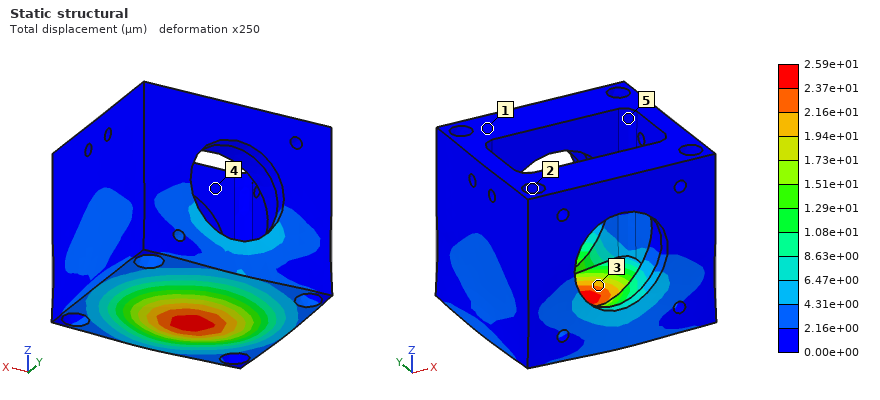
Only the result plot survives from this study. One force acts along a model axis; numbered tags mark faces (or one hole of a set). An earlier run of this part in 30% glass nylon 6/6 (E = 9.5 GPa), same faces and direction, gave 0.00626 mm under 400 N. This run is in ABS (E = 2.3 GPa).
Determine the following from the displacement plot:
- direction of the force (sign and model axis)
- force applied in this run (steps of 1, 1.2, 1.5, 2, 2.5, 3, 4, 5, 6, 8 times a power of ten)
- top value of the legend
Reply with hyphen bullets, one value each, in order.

- -Z
- 400 N
- 2.59e+01 µm
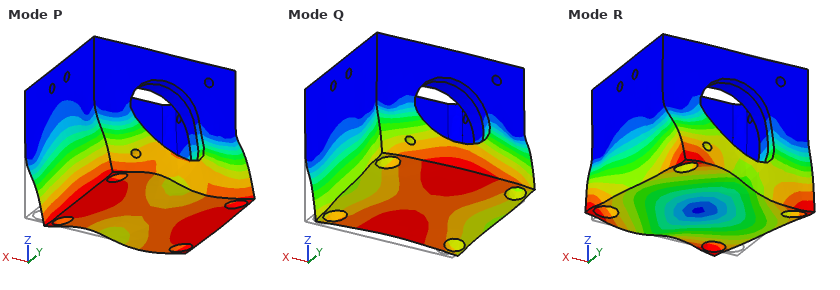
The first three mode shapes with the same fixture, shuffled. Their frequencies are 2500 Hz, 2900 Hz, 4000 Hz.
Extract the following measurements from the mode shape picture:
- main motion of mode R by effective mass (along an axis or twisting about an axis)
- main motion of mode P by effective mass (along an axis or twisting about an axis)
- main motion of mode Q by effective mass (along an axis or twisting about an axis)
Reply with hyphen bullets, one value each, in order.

- twisting about Z
- along X
- along Y
